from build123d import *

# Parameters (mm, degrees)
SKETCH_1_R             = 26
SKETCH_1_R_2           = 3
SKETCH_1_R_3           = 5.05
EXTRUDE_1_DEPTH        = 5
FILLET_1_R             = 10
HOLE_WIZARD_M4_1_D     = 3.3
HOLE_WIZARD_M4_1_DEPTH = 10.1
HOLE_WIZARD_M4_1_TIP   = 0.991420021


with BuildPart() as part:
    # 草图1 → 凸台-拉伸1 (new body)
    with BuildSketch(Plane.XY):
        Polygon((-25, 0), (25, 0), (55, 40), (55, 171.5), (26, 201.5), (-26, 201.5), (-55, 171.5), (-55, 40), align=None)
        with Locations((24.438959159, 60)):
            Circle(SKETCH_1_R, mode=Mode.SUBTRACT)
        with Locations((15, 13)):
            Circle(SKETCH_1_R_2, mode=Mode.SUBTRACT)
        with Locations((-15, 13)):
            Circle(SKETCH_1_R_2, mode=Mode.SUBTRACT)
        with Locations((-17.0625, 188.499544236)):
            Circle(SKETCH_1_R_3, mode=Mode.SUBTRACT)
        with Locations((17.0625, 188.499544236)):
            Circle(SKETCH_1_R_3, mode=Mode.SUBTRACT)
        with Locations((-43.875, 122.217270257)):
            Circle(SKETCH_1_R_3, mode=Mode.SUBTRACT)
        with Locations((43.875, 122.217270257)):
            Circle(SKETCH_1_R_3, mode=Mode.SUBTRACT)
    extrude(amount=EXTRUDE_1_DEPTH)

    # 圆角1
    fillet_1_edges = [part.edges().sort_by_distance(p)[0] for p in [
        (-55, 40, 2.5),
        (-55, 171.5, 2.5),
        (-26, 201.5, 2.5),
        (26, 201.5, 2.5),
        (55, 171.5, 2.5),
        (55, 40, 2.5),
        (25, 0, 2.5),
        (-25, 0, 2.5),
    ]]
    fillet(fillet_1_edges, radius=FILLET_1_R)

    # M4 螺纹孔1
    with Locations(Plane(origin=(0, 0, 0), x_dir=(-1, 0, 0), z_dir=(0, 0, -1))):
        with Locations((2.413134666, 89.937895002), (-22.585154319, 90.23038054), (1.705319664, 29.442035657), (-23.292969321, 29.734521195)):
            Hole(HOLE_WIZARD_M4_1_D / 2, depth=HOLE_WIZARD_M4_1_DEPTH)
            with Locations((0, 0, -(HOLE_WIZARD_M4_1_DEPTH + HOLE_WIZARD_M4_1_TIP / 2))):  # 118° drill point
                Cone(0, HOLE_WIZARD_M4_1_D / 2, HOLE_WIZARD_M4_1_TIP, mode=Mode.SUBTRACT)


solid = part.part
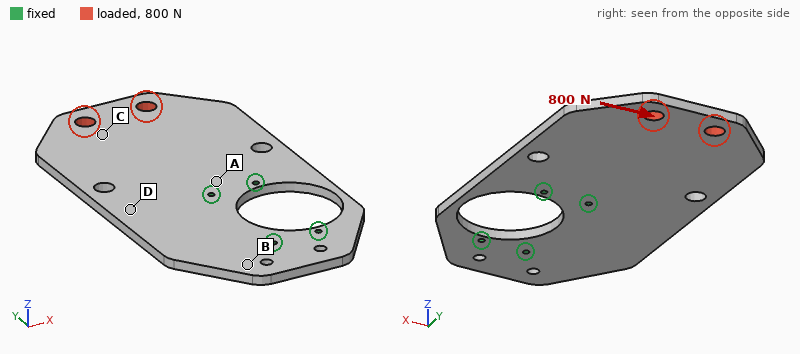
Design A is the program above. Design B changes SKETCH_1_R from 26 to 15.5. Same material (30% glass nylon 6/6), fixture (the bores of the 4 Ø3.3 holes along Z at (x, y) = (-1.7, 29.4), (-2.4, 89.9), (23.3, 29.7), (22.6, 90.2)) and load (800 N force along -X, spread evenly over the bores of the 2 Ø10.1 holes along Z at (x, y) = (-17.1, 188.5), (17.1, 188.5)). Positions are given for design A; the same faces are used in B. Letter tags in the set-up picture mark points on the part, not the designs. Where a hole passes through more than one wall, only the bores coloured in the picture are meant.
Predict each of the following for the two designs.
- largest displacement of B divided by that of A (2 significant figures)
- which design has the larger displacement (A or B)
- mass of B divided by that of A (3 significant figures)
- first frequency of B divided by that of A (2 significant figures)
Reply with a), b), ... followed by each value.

a) 0.83
b) A
c) 1.08
d) 1.0
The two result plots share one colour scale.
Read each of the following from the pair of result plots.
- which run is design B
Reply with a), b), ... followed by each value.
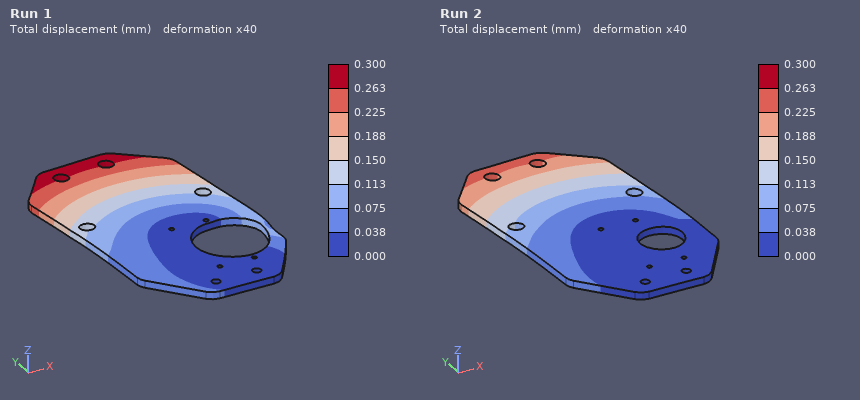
a) Run 2
